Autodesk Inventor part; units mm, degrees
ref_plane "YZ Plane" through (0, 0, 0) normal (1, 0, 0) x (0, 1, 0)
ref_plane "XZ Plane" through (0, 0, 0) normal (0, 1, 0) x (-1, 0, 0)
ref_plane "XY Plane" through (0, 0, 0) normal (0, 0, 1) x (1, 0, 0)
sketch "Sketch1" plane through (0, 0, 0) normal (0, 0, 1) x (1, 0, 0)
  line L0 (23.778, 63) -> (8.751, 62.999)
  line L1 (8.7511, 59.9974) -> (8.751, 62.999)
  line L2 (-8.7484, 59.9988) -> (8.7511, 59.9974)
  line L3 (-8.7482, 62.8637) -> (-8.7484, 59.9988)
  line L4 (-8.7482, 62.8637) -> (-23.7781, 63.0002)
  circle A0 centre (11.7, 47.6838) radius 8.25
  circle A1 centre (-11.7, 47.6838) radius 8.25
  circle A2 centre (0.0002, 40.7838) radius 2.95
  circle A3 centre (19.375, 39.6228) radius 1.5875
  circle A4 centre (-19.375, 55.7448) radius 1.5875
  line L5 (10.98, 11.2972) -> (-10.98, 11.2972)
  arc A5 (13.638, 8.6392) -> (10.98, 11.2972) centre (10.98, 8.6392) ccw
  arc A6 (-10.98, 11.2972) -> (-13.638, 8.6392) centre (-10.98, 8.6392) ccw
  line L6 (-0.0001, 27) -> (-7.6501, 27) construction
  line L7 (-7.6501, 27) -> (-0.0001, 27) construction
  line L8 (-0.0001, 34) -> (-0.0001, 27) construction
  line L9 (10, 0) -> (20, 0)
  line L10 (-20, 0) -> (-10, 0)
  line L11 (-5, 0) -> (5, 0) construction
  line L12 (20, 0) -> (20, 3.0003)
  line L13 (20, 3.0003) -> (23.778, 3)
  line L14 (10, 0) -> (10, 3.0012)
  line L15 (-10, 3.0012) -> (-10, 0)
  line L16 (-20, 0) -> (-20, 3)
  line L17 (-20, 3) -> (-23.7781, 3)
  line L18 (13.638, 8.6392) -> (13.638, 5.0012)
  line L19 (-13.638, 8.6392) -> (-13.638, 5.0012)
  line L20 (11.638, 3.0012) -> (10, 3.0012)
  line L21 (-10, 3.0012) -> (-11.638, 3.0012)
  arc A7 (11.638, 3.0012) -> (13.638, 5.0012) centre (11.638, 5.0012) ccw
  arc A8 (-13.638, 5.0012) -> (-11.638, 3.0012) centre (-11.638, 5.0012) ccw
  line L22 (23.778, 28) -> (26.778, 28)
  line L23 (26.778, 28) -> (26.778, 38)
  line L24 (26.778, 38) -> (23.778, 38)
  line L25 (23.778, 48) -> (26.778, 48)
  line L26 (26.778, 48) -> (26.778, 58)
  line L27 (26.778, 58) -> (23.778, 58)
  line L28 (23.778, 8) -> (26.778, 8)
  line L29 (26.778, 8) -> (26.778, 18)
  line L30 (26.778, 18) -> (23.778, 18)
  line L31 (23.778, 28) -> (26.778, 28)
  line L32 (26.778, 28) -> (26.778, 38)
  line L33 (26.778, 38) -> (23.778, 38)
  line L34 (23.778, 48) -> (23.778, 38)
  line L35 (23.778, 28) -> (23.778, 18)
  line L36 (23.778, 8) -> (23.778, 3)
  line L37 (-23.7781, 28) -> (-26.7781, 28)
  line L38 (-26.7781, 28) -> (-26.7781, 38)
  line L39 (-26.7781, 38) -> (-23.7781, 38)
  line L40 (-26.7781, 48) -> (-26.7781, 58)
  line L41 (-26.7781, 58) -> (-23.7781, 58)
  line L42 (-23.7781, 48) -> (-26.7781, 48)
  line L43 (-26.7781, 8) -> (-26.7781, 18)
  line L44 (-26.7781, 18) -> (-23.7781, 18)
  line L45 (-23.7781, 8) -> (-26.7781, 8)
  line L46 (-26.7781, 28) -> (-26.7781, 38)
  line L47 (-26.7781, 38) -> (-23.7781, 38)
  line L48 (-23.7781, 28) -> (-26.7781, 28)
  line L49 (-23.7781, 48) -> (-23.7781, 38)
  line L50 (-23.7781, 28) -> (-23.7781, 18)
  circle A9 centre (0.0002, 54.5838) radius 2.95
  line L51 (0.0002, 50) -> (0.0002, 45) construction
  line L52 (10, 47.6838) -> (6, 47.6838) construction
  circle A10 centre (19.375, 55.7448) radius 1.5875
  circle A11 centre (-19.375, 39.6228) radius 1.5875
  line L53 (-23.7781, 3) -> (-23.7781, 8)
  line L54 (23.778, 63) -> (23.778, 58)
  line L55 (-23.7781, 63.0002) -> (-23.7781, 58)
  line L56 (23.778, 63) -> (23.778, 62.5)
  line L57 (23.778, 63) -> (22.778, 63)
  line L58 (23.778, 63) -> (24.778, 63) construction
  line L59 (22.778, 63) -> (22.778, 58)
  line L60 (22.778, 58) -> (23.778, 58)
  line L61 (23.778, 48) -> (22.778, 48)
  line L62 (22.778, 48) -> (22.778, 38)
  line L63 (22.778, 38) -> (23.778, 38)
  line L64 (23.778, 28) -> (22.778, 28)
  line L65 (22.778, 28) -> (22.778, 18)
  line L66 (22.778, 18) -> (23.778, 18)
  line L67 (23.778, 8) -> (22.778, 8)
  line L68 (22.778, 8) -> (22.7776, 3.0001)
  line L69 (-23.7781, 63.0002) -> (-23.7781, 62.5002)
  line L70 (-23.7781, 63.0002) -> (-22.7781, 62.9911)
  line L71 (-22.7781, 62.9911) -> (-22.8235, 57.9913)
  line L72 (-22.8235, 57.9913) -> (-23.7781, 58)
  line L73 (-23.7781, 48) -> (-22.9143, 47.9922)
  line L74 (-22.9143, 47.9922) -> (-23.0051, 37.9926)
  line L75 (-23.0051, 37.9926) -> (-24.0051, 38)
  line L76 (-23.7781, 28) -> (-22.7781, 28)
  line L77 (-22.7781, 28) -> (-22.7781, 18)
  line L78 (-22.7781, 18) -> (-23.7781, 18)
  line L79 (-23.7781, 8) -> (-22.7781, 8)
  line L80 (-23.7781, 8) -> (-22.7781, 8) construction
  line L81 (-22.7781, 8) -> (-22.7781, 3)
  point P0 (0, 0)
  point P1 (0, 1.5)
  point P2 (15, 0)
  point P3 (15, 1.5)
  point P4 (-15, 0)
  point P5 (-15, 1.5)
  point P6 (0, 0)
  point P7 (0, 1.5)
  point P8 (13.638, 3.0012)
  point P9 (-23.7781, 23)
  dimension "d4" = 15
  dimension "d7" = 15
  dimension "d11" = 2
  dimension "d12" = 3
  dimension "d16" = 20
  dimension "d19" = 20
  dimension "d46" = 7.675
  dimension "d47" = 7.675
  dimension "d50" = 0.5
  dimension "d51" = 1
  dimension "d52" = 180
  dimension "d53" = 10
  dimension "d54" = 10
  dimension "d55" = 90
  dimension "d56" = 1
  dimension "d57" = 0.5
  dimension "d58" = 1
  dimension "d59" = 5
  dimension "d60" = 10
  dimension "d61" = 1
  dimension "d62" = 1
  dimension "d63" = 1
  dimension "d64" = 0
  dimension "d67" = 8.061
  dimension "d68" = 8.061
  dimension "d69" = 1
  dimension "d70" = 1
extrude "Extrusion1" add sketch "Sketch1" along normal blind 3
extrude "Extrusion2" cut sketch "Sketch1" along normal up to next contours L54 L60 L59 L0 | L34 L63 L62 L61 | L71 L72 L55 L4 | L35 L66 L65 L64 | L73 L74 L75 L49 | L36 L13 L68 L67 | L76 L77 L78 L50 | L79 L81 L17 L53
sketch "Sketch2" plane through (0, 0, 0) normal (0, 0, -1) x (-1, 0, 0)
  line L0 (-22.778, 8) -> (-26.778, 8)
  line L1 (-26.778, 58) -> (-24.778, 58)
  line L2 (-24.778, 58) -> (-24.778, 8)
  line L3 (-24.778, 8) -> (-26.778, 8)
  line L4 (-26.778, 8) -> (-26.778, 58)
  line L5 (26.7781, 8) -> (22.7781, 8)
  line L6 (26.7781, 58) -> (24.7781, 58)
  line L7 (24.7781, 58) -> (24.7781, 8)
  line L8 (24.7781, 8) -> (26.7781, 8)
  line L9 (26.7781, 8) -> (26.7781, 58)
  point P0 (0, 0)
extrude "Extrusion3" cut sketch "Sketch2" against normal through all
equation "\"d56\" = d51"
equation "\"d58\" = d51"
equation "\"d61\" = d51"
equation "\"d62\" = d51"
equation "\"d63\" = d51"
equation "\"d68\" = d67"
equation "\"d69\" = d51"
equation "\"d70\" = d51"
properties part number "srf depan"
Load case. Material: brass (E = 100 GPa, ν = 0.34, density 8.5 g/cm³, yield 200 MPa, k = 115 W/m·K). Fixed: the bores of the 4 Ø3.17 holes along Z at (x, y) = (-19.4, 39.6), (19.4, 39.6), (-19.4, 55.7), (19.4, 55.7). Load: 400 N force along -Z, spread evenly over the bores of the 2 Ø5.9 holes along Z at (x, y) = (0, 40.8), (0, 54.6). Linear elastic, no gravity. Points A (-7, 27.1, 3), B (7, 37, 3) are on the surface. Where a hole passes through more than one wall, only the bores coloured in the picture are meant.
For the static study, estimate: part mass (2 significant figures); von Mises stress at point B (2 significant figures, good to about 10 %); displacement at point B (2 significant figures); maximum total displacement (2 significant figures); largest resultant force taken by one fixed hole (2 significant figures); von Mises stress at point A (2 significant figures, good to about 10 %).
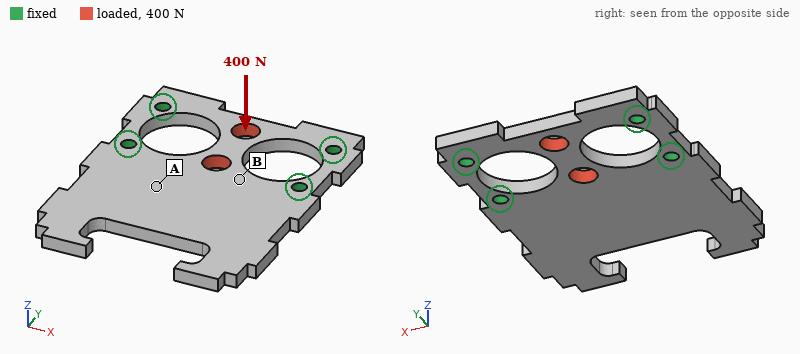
54 g
37 MPa
19 µm
45 µm
100 N
15 MPa
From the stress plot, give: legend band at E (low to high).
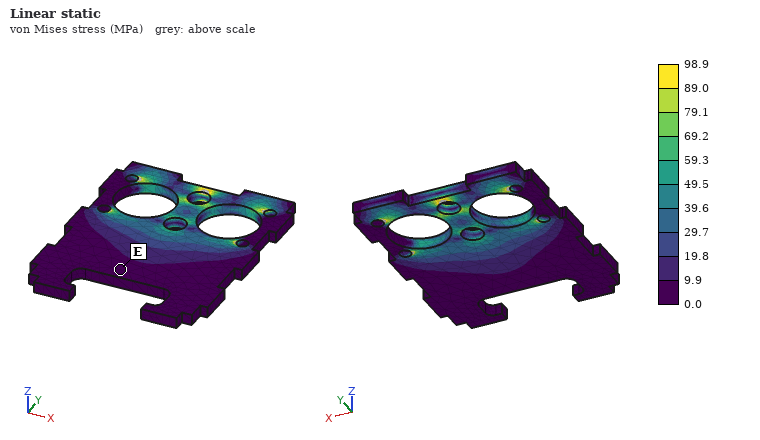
0.0 to 9.9 MPa
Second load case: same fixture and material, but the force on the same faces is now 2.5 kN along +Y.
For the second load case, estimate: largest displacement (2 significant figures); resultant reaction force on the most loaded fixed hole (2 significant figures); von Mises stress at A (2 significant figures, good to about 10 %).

30 µm
1.0 kN
26 MPa
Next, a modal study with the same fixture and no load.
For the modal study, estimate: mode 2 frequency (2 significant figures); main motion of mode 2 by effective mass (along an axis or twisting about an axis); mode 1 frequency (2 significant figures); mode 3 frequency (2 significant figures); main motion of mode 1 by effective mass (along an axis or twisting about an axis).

2100 Hz
twisting about Y
1100 Hz
4700 Hz
along Z
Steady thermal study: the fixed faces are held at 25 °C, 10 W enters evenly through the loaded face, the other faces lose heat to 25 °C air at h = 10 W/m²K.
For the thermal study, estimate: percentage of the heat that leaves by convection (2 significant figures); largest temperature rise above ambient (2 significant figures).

3.2 %
21 K
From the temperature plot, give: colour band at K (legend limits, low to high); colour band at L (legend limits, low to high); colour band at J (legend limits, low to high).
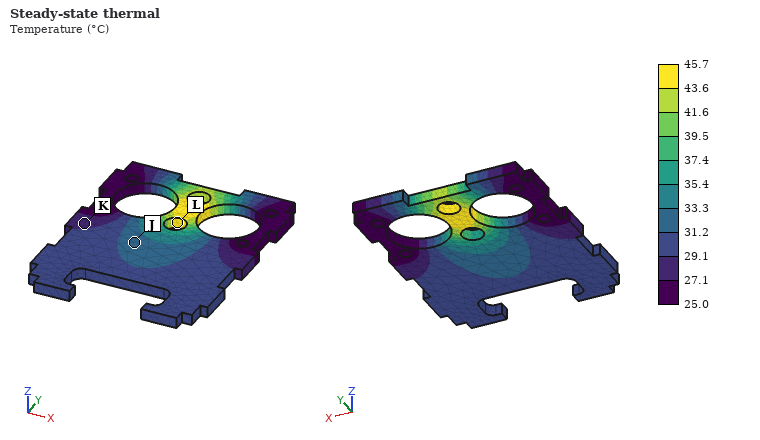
27.1 to 29.1 °C
43.6 to 45.7 °C
31.2 to 33.3 °C
